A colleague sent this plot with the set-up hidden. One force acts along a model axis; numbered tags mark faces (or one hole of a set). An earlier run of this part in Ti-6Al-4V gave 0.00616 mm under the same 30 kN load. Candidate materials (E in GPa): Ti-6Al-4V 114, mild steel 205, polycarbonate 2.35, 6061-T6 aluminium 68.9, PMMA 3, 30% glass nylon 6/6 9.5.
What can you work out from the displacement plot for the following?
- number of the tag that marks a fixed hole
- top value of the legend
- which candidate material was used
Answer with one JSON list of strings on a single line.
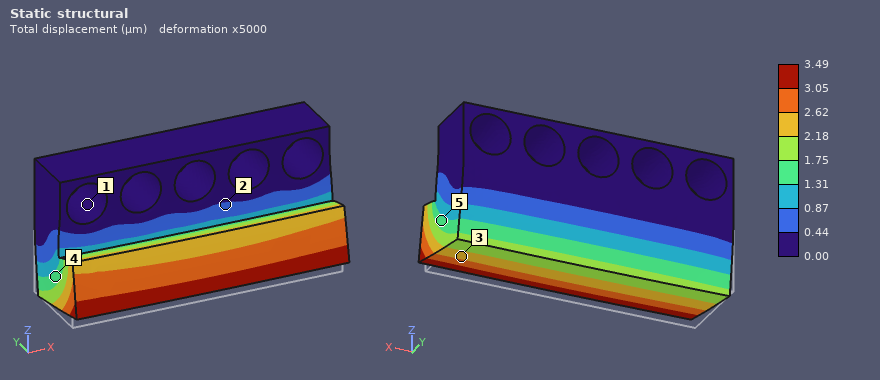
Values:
["1", "3.49 µm", "mild steel"]
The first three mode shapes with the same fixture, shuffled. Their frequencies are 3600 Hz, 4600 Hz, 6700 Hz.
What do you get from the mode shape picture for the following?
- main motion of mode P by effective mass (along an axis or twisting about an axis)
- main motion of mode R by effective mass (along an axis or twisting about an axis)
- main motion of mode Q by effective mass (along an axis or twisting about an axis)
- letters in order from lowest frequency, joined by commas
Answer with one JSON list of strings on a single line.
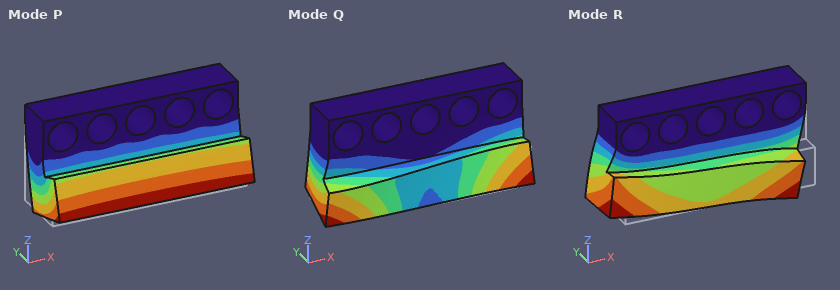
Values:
["along Y", "along X", "twisting about Z", "P, Q, R"]
